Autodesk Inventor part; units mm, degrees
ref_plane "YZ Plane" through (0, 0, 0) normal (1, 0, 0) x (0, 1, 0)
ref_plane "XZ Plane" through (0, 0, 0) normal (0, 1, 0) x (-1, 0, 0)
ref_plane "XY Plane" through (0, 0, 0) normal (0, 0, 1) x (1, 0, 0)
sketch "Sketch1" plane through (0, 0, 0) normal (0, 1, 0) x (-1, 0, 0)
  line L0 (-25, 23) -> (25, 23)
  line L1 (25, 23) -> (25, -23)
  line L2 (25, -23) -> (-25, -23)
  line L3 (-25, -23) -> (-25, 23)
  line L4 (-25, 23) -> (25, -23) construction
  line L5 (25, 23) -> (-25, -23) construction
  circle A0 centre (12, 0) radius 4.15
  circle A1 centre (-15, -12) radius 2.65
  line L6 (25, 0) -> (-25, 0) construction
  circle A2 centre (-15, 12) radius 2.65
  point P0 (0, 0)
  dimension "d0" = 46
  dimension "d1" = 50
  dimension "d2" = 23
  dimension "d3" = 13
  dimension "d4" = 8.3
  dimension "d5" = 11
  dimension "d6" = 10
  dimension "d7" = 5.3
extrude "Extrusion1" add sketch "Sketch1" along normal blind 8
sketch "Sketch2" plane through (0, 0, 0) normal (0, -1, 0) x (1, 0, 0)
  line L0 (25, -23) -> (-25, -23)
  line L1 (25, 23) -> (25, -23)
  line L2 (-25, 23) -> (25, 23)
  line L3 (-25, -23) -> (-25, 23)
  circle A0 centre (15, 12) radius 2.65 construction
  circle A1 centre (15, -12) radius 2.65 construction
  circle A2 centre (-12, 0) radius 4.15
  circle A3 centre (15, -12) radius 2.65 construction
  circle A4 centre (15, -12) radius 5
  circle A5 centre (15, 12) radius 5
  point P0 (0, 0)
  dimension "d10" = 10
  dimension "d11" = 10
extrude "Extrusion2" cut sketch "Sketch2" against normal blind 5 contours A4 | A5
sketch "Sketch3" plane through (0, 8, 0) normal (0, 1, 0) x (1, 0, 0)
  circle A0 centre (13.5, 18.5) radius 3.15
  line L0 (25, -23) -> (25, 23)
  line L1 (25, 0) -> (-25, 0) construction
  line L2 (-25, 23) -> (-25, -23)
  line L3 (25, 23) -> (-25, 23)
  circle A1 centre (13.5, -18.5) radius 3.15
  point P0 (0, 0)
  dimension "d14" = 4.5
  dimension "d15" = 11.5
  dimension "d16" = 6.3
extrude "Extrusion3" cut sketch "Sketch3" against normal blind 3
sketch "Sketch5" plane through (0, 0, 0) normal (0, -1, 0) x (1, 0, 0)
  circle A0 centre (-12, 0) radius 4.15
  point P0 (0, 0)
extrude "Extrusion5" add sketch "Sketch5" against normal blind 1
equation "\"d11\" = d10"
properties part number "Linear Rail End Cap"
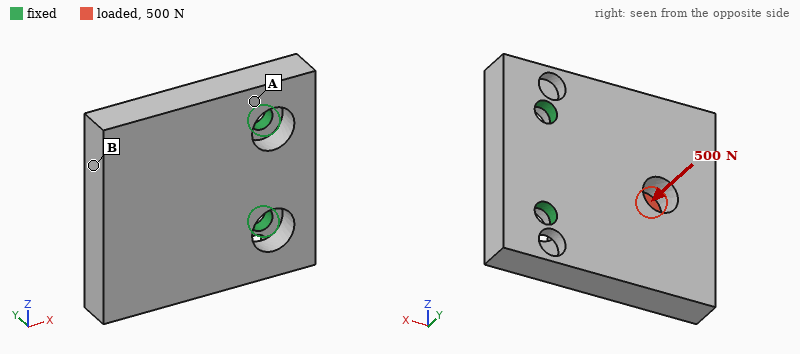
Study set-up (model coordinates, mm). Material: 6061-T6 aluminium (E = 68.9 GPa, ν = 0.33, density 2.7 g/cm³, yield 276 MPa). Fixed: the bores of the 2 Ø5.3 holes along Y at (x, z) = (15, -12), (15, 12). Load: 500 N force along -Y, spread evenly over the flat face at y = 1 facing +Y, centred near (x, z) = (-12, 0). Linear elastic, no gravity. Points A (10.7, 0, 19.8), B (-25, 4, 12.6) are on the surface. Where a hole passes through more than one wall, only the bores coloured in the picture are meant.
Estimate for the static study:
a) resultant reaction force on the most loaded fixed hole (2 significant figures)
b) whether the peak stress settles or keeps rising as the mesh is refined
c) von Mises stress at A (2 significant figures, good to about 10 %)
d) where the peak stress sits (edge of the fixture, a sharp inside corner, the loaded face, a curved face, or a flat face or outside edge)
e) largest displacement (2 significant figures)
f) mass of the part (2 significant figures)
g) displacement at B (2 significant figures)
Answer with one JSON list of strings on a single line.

["270 N", "keeps rising", "34 MPa", "edge of the fixture", "0.14 mm", "46 g", "0.13 mm"]
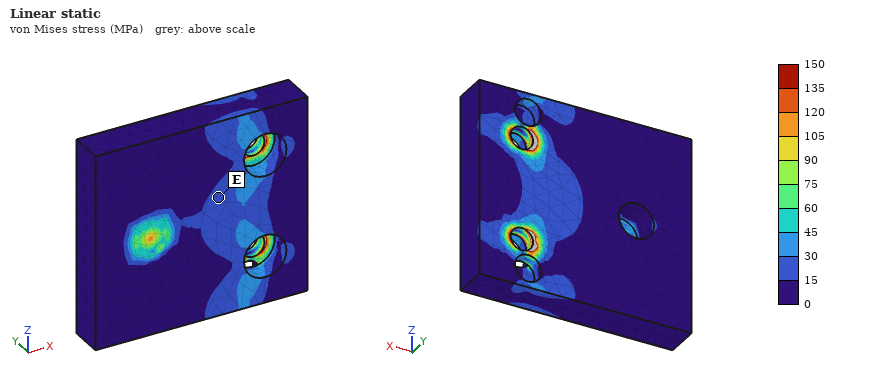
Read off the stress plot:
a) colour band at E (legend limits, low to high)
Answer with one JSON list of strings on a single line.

["15 to 30 MPa"]
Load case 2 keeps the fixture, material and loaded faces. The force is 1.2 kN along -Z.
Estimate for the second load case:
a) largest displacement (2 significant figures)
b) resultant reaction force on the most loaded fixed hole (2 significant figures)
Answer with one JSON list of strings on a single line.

["20 µm", "1.4 kN"]
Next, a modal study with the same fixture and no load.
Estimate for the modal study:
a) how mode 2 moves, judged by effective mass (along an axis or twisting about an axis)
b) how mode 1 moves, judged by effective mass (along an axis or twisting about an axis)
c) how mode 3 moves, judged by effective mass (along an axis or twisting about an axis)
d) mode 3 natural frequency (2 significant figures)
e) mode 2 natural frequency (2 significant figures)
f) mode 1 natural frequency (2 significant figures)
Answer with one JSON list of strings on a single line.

["twisting about X", "along Y", "along Z", "8900 Hz", "6200 Hz", "2300 Hz"]
